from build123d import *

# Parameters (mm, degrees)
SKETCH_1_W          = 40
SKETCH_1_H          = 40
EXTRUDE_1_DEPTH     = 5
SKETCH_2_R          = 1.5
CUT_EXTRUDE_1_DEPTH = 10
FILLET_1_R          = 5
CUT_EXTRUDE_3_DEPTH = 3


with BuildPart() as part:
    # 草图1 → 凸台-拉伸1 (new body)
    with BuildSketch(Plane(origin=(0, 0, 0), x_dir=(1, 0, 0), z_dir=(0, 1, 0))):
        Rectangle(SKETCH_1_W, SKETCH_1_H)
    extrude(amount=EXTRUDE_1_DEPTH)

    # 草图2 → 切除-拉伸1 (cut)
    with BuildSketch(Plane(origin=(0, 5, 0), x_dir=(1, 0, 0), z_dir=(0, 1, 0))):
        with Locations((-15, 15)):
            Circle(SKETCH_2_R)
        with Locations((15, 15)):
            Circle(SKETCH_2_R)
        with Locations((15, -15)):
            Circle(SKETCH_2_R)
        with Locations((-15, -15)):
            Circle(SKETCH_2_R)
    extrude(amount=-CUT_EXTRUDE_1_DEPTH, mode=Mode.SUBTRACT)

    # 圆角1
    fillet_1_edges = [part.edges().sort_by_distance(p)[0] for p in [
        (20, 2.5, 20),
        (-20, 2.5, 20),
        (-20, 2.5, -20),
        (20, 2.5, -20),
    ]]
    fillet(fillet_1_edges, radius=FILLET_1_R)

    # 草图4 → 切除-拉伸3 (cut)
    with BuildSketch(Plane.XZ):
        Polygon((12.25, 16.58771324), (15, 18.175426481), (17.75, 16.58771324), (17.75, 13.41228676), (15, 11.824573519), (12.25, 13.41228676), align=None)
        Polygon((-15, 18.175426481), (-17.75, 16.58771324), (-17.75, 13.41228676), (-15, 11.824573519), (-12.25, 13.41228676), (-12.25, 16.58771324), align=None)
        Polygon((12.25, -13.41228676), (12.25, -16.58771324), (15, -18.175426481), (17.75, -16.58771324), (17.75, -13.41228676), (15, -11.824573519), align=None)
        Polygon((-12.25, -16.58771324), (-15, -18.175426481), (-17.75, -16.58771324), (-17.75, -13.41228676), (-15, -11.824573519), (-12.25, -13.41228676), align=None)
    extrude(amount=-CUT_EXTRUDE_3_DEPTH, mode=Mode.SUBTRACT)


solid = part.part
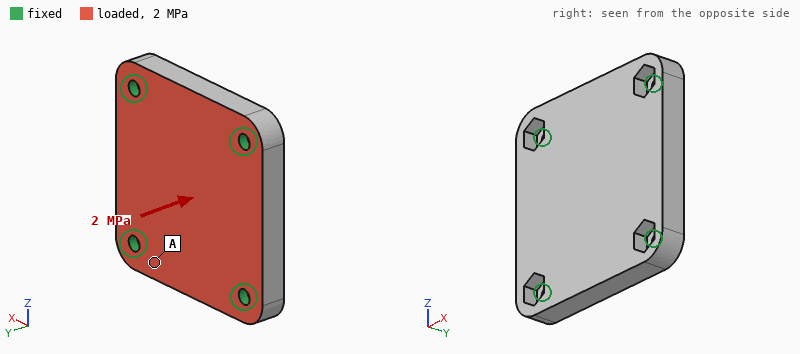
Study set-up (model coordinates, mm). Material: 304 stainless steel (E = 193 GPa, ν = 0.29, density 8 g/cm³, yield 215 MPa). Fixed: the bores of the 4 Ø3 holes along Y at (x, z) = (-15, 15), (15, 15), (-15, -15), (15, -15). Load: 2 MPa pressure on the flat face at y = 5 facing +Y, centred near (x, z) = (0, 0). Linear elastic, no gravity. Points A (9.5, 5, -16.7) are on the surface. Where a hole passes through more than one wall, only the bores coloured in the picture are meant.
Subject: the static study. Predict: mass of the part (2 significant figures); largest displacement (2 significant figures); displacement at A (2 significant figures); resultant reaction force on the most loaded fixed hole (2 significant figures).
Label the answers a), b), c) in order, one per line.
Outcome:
a) 60 g
b) 9.7 µm
c) 3.2 µm
d) 940 N
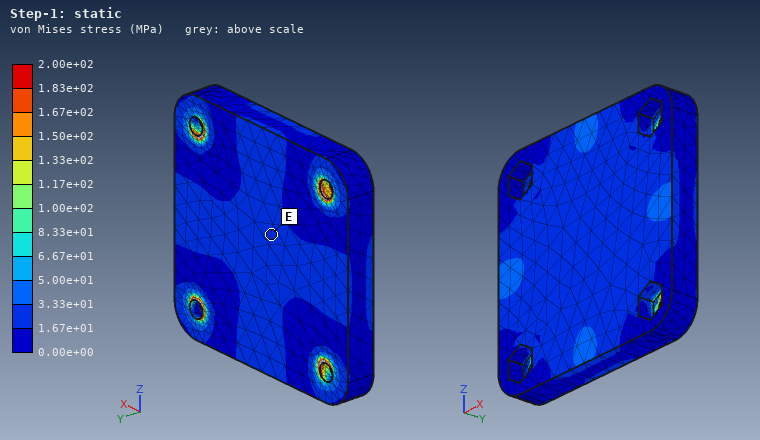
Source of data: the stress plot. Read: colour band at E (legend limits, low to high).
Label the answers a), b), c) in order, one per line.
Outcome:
a) 1.67e+01 to 3.33e+01 MPa
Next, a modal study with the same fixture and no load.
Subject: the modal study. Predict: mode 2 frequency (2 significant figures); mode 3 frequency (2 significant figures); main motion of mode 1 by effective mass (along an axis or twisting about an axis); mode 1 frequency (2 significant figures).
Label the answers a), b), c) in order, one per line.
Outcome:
a) 20 kHz
b) 20 kHz
c) along Y
d) 14 kHz
